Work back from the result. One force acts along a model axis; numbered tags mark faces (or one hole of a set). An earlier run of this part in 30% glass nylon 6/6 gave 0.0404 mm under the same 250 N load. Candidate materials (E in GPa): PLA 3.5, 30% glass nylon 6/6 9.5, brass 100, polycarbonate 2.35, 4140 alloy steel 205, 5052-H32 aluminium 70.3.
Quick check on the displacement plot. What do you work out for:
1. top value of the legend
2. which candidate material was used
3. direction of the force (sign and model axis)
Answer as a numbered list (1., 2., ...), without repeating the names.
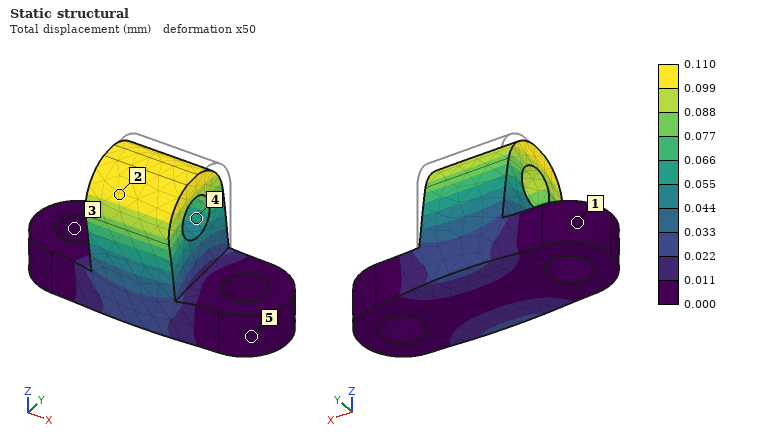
1. 0.110 mm
2. PLA
3. -Y
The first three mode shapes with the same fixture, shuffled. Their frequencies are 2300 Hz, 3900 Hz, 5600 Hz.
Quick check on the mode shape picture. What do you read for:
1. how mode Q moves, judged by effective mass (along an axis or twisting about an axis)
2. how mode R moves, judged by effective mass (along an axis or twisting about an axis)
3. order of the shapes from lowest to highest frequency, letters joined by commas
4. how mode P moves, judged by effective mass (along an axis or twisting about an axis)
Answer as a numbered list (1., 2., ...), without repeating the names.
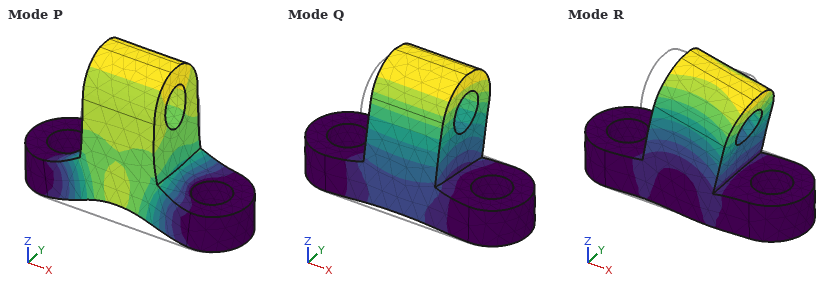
1. along Y
2. along X
3. Q, R, P
4. along Z
